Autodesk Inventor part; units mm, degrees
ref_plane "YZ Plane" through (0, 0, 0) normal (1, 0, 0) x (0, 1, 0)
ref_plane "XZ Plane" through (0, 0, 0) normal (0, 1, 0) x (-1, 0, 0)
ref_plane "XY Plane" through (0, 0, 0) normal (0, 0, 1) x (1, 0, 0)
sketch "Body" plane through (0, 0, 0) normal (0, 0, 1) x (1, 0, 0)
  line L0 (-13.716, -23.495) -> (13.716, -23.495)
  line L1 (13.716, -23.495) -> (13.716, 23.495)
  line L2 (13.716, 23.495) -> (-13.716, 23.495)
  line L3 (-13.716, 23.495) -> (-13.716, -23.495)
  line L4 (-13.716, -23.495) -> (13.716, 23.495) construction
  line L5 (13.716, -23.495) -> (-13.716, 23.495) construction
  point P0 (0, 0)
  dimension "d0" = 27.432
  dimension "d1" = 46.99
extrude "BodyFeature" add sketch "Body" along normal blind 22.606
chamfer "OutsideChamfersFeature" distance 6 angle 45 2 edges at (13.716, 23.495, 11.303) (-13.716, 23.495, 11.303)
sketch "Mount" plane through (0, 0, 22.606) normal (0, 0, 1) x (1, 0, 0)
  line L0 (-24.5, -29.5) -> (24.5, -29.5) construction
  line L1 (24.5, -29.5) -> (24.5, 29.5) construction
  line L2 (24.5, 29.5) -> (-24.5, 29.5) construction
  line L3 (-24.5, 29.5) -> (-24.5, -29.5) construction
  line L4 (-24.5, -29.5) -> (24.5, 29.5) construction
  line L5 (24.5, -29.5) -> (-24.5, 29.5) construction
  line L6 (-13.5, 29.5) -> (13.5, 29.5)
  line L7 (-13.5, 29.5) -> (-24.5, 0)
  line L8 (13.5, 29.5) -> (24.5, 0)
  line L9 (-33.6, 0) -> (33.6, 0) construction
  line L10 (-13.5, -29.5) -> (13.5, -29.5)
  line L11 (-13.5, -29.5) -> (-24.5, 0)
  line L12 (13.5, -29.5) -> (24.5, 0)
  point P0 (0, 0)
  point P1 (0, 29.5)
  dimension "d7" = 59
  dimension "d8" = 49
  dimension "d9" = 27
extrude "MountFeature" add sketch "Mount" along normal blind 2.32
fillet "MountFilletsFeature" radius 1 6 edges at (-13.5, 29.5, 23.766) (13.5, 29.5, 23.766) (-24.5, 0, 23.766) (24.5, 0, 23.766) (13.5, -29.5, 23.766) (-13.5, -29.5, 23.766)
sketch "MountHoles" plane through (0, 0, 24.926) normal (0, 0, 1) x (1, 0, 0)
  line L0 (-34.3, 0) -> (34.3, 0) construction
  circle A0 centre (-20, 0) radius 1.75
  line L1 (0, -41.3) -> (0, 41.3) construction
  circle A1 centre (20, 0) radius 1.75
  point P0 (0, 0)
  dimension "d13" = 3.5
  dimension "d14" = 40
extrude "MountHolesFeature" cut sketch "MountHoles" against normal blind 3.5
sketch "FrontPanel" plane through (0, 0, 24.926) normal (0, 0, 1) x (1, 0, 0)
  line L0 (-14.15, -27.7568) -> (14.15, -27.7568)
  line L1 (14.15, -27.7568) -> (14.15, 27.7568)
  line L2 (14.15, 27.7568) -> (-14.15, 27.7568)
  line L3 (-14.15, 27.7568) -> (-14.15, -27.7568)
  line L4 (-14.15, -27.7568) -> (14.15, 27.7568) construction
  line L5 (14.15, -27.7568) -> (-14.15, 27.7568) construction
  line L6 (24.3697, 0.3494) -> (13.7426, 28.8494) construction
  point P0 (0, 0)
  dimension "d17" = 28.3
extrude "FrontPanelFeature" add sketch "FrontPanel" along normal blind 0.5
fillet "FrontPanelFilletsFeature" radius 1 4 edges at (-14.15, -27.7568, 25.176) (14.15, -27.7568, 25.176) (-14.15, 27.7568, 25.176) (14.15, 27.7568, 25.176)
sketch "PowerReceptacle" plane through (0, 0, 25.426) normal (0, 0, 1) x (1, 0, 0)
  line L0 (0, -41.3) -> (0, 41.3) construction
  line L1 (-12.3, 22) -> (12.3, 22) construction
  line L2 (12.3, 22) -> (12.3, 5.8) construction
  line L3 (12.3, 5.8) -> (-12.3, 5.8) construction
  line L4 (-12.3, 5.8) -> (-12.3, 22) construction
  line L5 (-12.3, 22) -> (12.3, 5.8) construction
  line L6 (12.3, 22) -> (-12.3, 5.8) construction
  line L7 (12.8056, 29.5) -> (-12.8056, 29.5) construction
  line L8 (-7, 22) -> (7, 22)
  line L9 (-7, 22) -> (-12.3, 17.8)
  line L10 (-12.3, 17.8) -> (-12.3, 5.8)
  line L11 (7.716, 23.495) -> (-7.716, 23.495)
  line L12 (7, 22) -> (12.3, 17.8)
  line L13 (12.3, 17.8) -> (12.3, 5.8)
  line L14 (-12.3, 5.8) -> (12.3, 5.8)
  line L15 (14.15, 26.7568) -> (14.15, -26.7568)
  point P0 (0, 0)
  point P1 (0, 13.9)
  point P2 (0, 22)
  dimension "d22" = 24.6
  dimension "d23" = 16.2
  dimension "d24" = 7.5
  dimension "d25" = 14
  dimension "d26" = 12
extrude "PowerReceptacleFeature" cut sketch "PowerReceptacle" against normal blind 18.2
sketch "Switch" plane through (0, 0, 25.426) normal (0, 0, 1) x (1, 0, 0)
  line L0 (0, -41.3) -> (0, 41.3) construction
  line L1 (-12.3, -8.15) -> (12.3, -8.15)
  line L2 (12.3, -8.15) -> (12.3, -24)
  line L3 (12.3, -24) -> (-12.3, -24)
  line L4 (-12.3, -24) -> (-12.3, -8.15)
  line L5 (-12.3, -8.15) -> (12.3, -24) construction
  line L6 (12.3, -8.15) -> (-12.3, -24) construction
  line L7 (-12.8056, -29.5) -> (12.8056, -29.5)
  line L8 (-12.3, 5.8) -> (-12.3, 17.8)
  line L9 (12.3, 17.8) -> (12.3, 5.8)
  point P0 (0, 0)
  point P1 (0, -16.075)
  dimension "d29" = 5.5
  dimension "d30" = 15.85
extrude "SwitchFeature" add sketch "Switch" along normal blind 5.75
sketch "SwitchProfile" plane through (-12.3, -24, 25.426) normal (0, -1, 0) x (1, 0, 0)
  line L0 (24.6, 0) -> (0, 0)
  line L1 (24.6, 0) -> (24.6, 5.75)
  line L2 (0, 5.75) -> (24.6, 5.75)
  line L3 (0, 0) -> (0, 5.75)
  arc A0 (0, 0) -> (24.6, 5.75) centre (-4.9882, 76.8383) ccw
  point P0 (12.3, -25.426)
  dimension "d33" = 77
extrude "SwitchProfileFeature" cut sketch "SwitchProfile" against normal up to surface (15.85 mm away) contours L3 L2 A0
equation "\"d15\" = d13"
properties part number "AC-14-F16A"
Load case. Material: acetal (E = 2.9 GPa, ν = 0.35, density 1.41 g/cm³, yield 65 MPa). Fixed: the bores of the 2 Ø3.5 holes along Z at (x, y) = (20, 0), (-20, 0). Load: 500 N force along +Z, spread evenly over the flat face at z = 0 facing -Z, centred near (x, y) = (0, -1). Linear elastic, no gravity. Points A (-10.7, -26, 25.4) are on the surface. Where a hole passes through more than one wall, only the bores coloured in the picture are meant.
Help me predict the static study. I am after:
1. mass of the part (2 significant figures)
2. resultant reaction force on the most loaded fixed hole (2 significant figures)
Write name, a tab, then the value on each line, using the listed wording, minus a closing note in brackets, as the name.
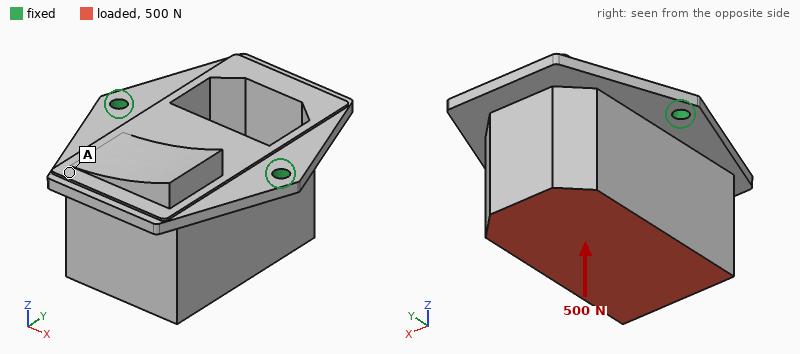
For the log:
mass of the part	40 g
resultant reaction force on the most loaded fixed hole	260 N
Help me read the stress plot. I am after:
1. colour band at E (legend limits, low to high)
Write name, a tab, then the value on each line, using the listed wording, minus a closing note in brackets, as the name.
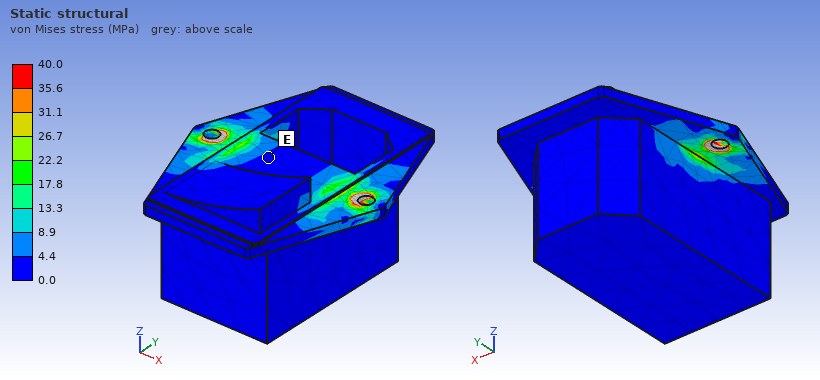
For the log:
colour band at E	0.0 to 4.4 MPa
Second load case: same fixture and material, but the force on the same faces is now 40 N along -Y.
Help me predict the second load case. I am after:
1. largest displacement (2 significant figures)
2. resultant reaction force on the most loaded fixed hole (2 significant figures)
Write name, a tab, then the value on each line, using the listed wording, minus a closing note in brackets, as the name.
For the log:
largest displacement	0.82 mm
resultant reaction force on the most loaded fixed hole	22 N
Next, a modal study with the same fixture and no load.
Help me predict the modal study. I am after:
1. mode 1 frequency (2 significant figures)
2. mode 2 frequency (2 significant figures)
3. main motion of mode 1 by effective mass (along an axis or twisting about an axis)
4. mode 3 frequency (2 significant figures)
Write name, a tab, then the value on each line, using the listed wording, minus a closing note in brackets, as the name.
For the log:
mode 1 frequency	260 Hz
mode 2 frequency	1300 Hz
main motion of mode 1 by effective mass	along Y
mode 3 frequency	1300 Hz
